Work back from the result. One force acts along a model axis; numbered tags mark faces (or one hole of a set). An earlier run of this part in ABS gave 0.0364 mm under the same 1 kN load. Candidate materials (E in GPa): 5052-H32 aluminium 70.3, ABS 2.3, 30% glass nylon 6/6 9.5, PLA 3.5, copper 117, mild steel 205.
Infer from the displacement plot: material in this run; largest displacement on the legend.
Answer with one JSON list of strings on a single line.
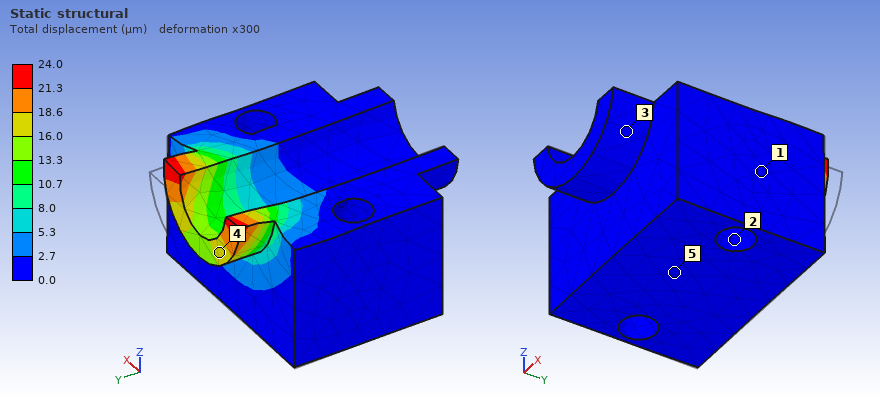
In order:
["PLA", "24.0 µm"]
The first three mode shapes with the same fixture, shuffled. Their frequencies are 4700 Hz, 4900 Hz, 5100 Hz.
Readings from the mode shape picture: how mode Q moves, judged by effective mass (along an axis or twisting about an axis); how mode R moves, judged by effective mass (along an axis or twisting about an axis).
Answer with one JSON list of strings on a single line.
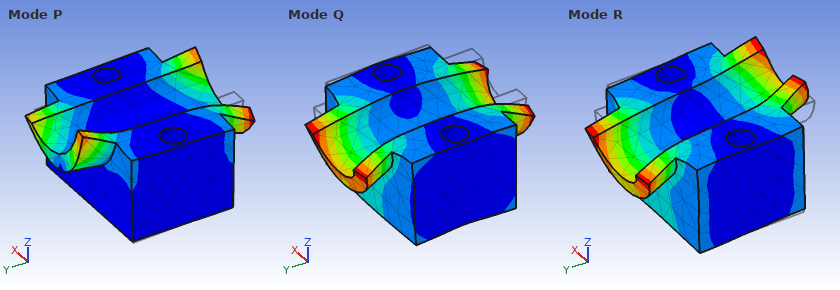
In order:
["along Z", "twisting about X"]
